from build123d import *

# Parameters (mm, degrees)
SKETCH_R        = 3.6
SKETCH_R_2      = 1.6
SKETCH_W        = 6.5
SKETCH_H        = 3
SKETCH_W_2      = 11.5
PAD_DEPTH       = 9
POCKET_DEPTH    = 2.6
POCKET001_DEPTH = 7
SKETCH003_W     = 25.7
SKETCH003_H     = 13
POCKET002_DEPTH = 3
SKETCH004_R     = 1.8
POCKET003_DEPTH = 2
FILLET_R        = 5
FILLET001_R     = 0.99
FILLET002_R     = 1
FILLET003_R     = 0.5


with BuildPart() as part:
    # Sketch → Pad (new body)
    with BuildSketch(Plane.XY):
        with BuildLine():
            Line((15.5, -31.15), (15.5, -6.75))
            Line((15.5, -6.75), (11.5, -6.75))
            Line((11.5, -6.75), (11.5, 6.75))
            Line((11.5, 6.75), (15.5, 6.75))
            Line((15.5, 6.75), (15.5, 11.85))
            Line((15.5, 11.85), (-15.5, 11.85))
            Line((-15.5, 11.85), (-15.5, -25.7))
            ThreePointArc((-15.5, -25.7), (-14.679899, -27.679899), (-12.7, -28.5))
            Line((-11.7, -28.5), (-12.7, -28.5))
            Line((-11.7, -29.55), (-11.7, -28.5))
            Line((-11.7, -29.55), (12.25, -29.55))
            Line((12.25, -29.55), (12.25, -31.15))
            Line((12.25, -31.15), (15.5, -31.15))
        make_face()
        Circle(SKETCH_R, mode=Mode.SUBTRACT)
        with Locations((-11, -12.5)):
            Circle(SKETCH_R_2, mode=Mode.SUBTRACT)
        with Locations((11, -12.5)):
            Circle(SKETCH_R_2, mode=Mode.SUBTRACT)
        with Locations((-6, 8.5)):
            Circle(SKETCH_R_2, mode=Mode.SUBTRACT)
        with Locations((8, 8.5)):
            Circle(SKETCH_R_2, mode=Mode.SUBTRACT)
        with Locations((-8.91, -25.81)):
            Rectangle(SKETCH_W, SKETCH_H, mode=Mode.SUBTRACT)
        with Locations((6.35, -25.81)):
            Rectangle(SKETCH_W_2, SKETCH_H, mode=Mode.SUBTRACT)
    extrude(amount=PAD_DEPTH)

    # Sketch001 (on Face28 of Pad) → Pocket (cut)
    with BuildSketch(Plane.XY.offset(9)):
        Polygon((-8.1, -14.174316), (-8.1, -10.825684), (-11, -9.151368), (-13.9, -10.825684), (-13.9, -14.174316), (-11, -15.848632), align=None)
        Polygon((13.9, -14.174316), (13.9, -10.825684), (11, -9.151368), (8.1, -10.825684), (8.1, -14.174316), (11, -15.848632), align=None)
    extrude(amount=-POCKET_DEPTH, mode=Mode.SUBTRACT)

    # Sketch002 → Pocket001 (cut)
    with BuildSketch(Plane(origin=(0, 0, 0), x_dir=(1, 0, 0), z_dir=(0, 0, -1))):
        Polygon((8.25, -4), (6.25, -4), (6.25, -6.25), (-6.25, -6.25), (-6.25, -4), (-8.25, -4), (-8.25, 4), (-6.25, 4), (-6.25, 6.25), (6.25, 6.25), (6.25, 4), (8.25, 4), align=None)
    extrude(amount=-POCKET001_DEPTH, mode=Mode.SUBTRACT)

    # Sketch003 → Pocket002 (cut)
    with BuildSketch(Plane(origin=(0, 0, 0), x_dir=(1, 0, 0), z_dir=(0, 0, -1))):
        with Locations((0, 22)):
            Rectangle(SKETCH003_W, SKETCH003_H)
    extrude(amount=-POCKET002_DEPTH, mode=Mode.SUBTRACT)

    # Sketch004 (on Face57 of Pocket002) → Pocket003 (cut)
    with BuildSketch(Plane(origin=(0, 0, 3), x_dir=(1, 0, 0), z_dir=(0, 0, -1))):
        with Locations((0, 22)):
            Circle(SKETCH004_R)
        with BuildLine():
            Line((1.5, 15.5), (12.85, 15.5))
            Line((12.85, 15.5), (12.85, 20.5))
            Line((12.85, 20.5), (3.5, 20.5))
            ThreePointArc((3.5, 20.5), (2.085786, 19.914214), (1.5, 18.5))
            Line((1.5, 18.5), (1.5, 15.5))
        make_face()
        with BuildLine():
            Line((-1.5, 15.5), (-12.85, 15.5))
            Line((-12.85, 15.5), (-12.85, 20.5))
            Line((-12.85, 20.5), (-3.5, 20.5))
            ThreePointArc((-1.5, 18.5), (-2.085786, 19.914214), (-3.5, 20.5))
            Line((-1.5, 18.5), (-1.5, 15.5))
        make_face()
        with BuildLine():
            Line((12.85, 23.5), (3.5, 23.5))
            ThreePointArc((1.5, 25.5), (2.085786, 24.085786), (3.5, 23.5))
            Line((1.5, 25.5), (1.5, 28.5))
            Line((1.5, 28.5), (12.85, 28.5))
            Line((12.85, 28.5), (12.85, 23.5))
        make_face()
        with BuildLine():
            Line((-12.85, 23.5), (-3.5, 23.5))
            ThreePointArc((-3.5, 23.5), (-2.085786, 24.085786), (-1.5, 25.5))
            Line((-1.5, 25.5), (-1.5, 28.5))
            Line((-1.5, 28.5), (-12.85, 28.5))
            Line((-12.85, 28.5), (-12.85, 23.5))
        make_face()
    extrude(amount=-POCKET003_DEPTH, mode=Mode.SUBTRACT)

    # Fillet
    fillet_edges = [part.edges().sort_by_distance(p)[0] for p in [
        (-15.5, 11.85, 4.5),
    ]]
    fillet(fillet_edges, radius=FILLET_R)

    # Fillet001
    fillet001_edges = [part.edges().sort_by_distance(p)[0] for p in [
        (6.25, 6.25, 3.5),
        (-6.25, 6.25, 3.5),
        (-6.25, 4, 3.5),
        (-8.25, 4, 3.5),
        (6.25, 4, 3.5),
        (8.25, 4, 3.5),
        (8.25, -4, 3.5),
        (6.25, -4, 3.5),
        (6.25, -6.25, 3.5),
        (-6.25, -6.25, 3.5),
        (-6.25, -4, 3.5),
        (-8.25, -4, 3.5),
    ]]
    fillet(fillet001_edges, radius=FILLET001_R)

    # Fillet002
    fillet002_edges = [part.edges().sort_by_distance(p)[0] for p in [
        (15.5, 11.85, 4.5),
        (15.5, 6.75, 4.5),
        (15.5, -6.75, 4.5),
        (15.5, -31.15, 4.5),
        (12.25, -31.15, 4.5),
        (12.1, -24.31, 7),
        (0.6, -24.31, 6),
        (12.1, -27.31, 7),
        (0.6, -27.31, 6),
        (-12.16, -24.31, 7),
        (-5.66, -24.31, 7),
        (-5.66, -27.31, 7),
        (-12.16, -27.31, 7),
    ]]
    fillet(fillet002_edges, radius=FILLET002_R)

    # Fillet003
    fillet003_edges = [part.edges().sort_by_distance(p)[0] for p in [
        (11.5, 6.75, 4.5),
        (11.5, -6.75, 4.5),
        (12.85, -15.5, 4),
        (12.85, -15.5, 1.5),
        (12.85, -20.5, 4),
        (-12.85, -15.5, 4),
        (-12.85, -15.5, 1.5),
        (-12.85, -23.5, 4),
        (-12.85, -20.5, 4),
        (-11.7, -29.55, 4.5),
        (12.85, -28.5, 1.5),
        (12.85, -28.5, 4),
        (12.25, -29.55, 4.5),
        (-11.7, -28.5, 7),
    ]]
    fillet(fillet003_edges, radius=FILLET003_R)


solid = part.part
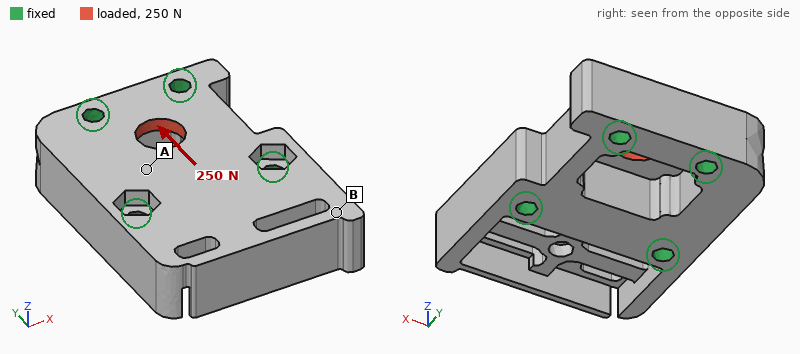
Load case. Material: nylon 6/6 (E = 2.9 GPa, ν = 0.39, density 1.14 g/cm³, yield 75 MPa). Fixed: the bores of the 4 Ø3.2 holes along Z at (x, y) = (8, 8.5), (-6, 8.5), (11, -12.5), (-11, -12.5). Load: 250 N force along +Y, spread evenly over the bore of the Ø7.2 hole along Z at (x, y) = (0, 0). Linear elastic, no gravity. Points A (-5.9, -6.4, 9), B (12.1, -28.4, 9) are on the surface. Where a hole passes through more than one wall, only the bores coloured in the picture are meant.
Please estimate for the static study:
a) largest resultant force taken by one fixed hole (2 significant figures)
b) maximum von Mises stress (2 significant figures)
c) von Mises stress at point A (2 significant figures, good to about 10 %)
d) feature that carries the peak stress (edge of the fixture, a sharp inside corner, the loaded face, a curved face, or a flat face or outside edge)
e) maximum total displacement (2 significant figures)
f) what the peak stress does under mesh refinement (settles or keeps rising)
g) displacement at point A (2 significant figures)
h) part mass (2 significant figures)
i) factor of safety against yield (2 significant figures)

87 N
10 MPa
2.7 MPa
the loaded face
21 µm
settles
8.4 µm
8.6 g
7.3
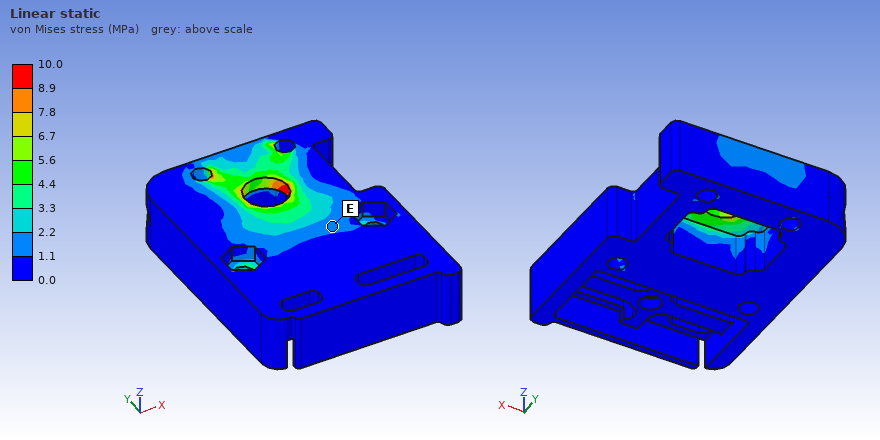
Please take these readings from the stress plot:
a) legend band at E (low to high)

1.1 to 2.2 MPa
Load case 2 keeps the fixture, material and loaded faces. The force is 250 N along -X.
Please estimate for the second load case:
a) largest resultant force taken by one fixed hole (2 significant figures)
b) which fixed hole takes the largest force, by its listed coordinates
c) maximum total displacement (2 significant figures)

77 N
(-6, 8.5)
21 µm
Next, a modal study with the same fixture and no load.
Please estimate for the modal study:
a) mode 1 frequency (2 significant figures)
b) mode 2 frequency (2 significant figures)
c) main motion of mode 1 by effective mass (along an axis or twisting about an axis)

4100 Hz
5600 Hz
along Z
